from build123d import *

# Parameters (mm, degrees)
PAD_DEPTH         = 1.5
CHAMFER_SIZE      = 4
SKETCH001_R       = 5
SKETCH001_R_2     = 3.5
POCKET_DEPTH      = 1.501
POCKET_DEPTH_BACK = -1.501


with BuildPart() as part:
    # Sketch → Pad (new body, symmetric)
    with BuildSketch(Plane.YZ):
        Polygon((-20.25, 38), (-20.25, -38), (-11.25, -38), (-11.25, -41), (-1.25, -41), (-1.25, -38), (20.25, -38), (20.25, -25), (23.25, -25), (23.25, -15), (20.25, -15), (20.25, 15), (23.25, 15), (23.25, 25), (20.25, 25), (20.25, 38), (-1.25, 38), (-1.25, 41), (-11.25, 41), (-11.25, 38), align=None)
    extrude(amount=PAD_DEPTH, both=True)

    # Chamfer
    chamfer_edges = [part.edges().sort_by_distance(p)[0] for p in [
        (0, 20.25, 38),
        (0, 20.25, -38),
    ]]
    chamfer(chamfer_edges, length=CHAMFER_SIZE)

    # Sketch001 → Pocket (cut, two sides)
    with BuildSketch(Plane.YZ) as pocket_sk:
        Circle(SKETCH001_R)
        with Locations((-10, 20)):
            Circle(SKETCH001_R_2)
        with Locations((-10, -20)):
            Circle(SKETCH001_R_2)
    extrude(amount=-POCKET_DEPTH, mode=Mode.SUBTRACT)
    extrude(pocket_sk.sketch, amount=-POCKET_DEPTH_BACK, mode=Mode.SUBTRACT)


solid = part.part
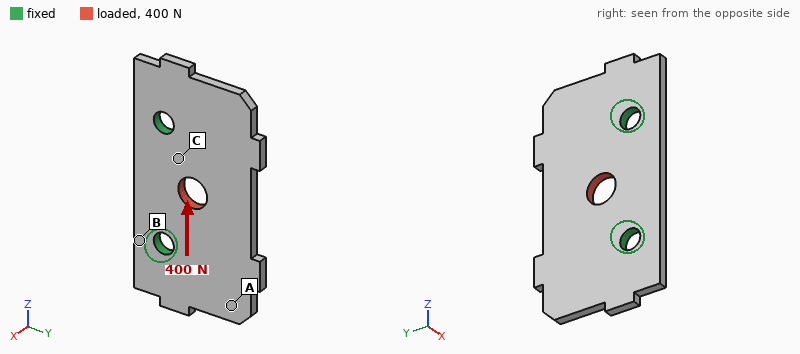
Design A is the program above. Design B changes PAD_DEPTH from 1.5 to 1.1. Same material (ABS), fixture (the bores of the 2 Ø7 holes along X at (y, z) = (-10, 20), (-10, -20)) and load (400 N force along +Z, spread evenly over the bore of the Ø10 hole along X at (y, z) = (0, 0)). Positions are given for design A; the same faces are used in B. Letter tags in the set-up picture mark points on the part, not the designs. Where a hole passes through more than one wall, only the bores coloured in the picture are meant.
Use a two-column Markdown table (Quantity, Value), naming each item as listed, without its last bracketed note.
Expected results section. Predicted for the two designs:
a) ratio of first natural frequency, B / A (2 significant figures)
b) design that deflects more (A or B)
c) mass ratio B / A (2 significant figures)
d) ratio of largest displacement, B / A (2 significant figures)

| Quantity | Value |
|---|---|
| ratio of first natural frequency, B / A | 0.75 |
| design that deflects more | B |
| mass ratio B / A | 0.73 |
| ratio of largest displacement, B / A | 1.4 |
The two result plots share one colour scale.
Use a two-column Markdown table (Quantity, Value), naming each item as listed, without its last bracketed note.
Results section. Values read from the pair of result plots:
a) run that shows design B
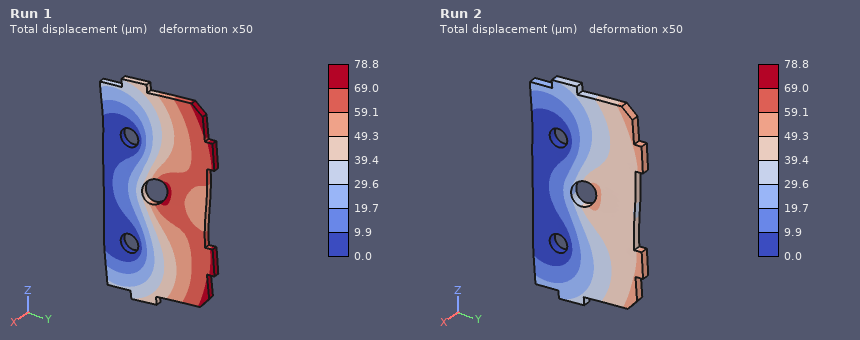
| Quantity | Value |
|---|---|
| run that shows design B | Run 1 |
